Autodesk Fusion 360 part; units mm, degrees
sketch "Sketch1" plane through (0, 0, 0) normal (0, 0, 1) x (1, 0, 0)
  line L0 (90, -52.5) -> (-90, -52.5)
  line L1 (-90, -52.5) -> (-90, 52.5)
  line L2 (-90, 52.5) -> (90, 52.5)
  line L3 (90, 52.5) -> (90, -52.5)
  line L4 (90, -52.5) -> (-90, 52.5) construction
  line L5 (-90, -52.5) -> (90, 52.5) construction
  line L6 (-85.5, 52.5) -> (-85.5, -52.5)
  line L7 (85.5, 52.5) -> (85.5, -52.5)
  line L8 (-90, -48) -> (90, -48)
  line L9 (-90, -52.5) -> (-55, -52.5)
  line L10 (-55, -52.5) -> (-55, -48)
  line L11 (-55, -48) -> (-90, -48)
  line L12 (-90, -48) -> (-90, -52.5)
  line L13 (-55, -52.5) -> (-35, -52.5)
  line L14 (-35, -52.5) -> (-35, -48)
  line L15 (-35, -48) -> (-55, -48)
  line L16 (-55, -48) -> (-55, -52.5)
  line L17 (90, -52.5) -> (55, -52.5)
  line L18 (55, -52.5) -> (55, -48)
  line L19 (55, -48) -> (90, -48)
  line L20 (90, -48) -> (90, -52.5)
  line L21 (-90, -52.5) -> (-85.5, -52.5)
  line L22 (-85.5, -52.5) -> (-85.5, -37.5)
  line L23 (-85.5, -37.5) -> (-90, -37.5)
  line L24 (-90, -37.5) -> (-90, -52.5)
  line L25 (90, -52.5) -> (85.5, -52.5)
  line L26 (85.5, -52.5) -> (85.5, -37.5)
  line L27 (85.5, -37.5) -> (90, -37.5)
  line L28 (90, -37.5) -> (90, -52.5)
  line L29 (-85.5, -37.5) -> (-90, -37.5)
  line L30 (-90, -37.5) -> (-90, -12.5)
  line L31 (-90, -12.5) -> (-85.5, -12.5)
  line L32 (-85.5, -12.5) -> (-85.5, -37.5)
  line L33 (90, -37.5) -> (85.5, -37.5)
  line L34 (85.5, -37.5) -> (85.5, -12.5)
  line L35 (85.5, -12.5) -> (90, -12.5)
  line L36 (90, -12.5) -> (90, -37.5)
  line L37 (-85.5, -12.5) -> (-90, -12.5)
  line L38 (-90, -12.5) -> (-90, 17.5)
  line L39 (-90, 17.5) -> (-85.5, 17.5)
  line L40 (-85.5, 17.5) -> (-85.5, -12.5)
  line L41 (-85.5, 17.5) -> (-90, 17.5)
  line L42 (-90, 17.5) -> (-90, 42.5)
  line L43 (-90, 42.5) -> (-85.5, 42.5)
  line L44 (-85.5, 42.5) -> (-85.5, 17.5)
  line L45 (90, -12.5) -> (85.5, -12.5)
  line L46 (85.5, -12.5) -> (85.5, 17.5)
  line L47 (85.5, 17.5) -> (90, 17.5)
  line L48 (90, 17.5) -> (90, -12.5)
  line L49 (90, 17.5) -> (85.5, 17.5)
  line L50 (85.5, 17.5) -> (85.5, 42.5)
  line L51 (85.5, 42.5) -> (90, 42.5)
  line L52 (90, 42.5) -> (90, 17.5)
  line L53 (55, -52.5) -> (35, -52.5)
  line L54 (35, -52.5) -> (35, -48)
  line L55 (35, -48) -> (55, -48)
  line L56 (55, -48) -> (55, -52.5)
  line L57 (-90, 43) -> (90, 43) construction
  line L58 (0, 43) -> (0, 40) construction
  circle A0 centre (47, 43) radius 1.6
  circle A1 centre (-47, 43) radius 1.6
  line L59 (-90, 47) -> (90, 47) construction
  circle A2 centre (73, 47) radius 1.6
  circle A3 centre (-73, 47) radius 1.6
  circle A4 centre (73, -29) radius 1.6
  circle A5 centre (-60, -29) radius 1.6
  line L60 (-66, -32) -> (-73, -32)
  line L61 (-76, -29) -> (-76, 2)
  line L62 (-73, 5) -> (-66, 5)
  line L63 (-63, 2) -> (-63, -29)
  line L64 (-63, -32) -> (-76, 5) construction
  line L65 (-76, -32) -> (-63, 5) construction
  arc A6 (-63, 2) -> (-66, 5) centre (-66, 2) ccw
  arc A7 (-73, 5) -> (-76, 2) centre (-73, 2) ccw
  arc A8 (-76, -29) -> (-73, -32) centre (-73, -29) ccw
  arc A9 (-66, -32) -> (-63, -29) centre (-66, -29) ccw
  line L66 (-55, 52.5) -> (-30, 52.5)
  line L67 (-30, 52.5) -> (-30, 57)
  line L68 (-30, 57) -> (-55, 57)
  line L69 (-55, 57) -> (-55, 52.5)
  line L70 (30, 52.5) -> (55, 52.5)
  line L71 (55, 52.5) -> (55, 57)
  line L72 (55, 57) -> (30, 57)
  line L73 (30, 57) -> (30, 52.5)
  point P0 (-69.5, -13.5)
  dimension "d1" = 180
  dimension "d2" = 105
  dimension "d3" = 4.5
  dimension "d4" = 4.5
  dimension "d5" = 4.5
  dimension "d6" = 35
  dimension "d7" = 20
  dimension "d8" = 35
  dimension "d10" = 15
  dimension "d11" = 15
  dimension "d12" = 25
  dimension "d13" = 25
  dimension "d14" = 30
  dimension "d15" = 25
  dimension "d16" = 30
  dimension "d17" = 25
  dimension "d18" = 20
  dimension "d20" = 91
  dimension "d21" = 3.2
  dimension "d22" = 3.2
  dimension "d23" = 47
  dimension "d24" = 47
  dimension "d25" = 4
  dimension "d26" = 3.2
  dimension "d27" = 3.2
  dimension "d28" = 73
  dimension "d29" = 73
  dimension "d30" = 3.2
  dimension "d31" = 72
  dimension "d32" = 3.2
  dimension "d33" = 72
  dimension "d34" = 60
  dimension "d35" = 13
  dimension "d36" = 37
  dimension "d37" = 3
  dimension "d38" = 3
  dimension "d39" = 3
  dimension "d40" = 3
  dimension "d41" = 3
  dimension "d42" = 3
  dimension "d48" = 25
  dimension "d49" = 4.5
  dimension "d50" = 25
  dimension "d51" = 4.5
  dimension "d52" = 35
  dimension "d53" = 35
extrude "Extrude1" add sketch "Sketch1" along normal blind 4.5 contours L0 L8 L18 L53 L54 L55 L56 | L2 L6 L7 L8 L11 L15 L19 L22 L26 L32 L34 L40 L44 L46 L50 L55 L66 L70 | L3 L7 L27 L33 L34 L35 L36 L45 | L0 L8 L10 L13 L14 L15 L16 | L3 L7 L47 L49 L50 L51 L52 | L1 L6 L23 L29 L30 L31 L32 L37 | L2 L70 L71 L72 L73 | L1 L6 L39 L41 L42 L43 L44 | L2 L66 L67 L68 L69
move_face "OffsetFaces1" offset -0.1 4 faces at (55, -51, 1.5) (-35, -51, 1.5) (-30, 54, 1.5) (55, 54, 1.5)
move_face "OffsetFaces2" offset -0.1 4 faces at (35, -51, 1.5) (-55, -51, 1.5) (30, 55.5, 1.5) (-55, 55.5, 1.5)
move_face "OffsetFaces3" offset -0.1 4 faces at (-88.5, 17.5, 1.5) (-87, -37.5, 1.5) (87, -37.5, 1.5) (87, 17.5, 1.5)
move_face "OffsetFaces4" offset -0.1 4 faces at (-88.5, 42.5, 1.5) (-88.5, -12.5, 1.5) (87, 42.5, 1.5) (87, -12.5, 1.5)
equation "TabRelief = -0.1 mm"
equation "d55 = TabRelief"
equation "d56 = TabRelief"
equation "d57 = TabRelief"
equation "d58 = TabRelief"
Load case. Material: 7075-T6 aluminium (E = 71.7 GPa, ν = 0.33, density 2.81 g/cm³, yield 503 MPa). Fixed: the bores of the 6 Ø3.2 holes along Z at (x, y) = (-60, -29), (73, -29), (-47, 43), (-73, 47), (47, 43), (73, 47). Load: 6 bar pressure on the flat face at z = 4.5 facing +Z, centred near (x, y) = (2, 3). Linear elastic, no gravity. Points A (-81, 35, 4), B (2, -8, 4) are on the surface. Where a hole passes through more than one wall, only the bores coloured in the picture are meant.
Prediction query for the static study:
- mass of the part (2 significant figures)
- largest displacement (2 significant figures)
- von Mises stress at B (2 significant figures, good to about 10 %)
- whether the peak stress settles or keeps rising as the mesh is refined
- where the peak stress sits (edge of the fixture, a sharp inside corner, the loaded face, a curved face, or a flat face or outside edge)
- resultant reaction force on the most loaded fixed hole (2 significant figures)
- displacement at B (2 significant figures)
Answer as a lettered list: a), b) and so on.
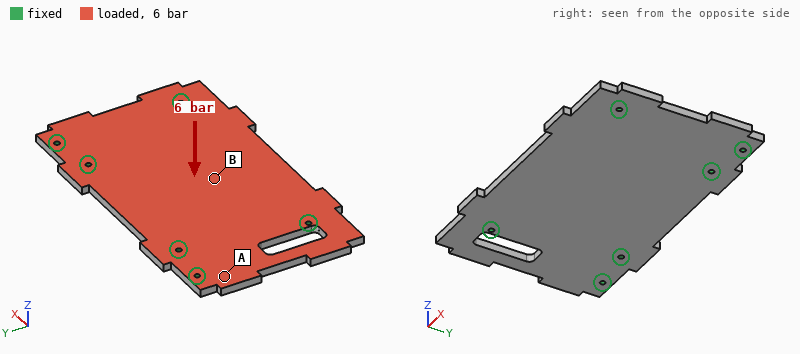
a) 220 g
b) 1.2 mm
c) 100 MPa
d) keeps rising
e) edge of the fixture
f) 2.8 kN
g) 0.87 mm
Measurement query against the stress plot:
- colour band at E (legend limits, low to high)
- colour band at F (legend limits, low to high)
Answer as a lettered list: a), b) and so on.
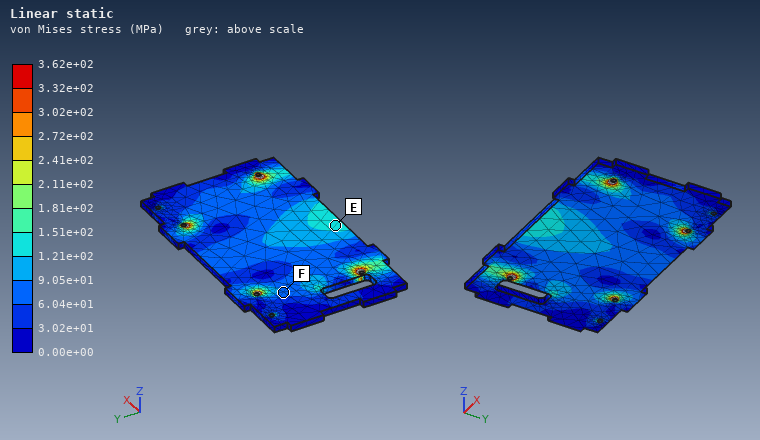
a) 1.21e+02 to 1.51e+02 MPa
b) 6.04e+01 to 9.05e+01 MPa
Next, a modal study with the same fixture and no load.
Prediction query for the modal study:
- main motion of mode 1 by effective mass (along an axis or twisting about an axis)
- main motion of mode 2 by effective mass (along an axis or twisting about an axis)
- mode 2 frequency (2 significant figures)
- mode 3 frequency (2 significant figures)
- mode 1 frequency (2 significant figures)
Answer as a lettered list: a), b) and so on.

a) along Z
b) along Z
c) 2300 Hz
d) 2500 Hz
e) 1300 Hz
